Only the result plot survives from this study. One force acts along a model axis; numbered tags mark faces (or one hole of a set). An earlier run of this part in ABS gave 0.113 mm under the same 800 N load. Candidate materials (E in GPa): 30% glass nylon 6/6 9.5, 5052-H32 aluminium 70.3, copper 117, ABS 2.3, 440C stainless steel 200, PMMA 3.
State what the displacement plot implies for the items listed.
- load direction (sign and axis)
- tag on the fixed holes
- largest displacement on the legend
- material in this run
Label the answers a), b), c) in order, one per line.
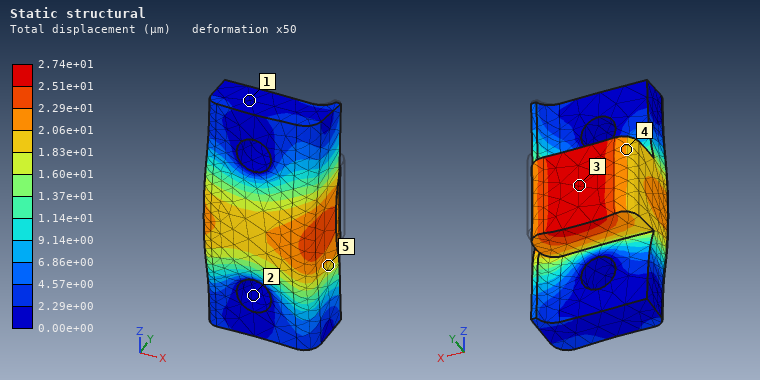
a) -Y
b) 2
c) 2.74e+01 µm
d) 30% glass nylon 6/6
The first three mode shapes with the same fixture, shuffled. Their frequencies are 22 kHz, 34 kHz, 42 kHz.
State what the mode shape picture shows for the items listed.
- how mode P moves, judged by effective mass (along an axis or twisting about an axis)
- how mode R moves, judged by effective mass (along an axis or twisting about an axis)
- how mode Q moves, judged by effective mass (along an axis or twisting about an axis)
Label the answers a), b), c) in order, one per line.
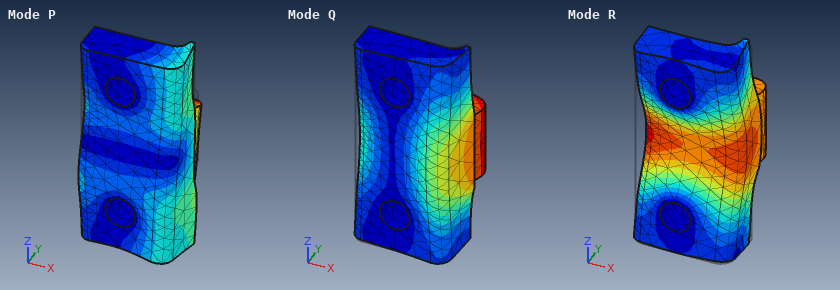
a) along Z
b) along Y
c) along X
